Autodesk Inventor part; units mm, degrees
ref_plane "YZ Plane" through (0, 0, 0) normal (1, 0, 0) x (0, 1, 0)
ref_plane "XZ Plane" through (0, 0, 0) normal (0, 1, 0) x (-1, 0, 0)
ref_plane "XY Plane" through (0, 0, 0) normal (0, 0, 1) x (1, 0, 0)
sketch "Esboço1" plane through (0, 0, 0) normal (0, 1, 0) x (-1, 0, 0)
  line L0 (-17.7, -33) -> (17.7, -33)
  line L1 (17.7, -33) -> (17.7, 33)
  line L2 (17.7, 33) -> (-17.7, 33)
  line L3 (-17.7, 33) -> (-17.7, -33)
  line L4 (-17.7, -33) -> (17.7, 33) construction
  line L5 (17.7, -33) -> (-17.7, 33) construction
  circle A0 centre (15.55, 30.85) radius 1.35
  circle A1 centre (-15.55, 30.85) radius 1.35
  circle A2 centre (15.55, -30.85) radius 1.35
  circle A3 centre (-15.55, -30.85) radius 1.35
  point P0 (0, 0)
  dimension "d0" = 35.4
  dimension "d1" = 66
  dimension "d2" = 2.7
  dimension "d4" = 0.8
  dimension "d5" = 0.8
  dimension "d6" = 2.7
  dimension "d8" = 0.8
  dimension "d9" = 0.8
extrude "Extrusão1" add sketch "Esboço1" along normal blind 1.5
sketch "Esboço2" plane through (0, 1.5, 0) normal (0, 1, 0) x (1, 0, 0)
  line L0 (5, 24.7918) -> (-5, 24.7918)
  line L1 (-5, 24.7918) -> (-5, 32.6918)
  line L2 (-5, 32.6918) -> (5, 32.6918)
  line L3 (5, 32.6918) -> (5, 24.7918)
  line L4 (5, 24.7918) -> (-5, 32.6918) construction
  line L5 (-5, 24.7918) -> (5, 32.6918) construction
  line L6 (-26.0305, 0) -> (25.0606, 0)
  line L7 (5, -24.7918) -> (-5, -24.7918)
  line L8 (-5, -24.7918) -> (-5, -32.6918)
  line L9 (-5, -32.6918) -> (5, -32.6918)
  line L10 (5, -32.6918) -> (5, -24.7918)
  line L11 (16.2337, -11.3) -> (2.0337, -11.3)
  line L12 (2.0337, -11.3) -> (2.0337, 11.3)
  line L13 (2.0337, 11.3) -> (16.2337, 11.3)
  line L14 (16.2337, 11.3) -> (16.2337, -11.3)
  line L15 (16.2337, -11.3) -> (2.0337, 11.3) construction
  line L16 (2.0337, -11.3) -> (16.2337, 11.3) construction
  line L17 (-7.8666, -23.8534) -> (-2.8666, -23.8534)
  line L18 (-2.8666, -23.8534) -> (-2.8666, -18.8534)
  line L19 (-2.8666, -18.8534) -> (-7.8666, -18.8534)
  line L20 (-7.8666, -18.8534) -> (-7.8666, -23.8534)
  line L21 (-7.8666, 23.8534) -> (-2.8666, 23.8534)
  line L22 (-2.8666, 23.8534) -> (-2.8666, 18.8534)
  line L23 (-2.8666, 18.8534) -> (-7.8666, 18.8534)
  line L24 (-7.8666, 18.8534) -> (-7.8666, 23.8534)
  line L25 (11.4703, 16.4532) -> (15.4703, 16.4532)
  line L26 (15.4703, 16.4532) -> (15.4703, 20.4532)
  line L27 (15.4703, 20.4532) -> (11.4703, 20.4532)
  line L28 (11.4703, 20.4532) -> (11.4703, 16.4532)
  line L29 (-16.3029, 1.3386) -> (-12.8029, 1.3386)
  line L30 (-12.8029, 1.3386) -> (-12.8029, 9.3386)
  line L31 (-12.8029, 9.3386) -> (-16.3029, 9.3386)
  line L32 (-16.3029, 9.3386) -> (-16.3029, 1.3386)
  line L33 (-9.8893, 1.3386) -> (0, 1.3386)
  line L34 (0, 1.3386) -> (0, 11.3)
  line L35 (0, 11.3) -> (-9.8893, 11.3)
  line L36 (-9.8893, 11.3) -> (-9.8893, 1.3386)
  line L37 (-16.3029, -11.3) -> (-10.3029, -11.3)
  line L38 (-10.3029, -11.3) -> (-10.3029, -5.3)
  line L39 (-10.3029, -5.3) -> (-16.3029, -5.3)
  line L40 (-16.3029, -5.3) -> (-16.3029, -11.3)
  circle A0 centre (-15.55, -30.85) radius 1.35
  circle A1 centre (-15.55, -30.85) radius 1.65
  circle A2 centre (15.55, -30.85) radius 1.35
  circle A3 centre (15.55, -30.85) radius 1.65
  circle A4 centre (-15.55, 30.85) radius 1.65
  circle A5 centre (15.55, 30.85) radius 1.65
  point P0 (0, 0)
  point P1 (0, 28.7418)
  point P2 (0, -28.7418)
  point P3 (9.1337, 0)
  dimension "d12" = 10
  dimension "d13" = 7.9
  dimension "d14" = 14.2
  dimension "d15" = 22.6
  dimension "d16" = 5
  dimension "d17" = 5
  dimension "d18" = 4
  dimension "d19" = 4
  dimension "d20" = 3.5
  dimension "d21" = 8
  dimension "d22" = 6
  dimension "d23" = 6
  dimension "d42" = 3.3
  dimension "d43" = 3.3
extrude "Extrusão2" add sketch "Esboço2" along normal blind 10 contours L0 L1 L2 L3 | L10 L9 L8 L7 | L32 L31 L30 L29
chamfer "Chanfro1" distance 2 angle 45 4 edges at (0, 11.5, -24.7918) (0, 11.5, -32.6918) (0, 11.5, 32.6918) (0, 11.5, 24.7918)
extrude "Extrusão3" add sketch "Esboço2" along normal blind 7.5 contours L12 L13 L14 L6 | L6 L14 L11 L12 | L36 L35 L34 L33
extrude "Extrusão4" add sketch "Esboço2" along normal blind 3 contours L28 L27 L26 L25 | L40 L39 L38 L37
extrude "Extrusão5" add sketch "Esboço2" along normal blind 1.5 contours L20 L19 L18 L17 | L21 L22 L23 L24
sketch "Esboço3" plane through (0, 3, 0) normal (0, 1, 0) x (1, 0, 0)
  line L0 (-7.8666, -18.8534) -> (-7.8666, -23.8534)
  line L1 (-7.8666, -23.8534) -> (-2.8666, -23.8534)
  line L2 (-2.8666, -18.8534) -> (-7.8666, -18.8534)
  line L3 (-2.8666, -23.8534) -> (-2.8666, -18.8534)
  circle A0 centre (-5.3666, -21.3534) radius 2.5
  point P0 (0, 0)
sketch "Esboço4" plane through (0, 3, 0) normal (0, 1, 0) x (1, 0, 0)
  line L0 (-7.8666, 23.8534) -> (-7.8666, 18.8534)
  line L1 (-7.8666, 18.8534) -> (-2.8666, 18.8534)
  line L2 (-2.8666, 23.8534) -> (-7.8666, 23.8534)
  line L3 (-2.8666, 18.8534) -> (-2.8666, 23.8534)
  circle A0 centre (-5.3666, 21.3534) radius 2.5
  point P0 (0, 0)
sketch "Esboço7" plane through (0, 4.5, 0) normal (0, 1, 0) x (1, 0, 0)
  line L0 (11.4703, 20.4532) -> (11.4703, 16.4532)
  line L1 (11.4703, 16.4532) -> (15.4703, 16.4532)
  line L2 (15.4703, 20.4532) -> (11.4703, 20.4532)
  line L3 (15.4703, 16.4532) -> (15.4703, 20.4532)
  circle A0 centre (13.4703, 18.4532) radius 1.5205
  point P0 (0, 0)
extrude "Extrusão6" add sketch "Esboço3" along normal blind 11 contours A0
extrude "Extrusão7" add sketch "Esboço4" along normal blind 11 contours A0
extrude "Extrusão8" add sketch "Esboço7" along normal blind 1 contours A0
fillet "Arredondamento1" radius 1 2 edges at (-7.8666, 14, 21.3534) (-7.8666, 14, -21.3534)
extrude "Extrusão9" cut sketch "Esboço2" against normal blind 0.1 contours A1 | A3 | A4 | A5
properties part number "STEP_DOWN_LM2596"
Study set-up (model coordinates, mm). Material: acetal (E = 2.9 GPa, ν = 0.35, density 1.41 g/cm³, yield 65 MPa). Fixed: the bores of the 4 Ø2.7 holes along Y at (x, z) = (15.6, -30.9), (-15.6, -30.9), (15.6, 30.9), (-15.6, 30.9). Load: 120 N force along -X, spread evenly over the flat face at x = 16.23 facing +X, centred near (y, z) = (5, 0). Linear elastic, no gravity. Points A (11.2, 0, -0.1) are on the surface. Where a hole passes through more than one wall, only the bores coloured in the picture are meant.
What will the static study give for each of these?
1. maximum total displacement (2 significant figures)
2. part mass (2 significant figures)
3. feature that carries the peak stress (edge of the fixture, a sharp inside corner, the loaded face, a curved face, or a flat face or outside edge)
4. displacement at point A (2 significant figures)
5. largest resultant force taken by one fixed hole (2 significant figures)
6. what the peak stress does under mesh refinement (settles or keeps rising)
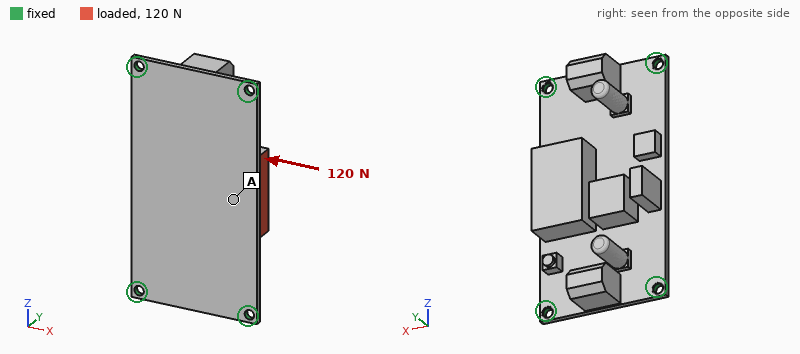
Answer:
0.78 mm
13 g
edge of the fixture
0.34 mm
46 N
keeps rising
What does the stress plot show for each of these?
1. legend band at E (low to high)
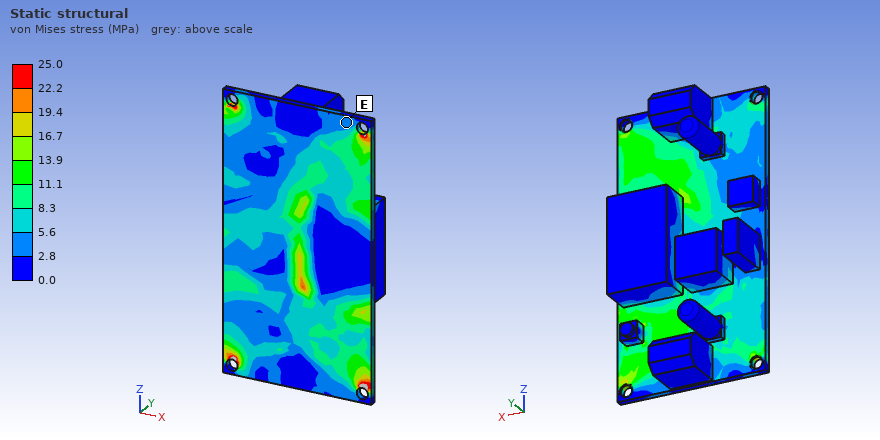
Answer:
2.8 to 5.6 MPa
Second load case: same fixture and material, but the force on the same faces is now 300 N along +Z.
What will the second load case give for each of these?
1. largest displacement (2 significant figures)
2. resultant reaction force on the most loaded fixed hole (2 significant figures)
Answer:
0.72 mm
94 N
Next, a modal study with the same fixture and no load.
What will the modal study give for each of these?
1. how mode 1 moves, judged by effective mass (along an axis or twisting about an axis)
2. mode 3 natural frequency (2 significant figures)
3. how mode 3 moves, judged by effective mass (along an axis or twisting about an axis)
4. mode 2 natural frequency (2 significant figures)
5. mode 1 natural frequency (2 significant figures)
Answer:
along Y
990 Hz
twisting about X
640 Hz
410 Hz
